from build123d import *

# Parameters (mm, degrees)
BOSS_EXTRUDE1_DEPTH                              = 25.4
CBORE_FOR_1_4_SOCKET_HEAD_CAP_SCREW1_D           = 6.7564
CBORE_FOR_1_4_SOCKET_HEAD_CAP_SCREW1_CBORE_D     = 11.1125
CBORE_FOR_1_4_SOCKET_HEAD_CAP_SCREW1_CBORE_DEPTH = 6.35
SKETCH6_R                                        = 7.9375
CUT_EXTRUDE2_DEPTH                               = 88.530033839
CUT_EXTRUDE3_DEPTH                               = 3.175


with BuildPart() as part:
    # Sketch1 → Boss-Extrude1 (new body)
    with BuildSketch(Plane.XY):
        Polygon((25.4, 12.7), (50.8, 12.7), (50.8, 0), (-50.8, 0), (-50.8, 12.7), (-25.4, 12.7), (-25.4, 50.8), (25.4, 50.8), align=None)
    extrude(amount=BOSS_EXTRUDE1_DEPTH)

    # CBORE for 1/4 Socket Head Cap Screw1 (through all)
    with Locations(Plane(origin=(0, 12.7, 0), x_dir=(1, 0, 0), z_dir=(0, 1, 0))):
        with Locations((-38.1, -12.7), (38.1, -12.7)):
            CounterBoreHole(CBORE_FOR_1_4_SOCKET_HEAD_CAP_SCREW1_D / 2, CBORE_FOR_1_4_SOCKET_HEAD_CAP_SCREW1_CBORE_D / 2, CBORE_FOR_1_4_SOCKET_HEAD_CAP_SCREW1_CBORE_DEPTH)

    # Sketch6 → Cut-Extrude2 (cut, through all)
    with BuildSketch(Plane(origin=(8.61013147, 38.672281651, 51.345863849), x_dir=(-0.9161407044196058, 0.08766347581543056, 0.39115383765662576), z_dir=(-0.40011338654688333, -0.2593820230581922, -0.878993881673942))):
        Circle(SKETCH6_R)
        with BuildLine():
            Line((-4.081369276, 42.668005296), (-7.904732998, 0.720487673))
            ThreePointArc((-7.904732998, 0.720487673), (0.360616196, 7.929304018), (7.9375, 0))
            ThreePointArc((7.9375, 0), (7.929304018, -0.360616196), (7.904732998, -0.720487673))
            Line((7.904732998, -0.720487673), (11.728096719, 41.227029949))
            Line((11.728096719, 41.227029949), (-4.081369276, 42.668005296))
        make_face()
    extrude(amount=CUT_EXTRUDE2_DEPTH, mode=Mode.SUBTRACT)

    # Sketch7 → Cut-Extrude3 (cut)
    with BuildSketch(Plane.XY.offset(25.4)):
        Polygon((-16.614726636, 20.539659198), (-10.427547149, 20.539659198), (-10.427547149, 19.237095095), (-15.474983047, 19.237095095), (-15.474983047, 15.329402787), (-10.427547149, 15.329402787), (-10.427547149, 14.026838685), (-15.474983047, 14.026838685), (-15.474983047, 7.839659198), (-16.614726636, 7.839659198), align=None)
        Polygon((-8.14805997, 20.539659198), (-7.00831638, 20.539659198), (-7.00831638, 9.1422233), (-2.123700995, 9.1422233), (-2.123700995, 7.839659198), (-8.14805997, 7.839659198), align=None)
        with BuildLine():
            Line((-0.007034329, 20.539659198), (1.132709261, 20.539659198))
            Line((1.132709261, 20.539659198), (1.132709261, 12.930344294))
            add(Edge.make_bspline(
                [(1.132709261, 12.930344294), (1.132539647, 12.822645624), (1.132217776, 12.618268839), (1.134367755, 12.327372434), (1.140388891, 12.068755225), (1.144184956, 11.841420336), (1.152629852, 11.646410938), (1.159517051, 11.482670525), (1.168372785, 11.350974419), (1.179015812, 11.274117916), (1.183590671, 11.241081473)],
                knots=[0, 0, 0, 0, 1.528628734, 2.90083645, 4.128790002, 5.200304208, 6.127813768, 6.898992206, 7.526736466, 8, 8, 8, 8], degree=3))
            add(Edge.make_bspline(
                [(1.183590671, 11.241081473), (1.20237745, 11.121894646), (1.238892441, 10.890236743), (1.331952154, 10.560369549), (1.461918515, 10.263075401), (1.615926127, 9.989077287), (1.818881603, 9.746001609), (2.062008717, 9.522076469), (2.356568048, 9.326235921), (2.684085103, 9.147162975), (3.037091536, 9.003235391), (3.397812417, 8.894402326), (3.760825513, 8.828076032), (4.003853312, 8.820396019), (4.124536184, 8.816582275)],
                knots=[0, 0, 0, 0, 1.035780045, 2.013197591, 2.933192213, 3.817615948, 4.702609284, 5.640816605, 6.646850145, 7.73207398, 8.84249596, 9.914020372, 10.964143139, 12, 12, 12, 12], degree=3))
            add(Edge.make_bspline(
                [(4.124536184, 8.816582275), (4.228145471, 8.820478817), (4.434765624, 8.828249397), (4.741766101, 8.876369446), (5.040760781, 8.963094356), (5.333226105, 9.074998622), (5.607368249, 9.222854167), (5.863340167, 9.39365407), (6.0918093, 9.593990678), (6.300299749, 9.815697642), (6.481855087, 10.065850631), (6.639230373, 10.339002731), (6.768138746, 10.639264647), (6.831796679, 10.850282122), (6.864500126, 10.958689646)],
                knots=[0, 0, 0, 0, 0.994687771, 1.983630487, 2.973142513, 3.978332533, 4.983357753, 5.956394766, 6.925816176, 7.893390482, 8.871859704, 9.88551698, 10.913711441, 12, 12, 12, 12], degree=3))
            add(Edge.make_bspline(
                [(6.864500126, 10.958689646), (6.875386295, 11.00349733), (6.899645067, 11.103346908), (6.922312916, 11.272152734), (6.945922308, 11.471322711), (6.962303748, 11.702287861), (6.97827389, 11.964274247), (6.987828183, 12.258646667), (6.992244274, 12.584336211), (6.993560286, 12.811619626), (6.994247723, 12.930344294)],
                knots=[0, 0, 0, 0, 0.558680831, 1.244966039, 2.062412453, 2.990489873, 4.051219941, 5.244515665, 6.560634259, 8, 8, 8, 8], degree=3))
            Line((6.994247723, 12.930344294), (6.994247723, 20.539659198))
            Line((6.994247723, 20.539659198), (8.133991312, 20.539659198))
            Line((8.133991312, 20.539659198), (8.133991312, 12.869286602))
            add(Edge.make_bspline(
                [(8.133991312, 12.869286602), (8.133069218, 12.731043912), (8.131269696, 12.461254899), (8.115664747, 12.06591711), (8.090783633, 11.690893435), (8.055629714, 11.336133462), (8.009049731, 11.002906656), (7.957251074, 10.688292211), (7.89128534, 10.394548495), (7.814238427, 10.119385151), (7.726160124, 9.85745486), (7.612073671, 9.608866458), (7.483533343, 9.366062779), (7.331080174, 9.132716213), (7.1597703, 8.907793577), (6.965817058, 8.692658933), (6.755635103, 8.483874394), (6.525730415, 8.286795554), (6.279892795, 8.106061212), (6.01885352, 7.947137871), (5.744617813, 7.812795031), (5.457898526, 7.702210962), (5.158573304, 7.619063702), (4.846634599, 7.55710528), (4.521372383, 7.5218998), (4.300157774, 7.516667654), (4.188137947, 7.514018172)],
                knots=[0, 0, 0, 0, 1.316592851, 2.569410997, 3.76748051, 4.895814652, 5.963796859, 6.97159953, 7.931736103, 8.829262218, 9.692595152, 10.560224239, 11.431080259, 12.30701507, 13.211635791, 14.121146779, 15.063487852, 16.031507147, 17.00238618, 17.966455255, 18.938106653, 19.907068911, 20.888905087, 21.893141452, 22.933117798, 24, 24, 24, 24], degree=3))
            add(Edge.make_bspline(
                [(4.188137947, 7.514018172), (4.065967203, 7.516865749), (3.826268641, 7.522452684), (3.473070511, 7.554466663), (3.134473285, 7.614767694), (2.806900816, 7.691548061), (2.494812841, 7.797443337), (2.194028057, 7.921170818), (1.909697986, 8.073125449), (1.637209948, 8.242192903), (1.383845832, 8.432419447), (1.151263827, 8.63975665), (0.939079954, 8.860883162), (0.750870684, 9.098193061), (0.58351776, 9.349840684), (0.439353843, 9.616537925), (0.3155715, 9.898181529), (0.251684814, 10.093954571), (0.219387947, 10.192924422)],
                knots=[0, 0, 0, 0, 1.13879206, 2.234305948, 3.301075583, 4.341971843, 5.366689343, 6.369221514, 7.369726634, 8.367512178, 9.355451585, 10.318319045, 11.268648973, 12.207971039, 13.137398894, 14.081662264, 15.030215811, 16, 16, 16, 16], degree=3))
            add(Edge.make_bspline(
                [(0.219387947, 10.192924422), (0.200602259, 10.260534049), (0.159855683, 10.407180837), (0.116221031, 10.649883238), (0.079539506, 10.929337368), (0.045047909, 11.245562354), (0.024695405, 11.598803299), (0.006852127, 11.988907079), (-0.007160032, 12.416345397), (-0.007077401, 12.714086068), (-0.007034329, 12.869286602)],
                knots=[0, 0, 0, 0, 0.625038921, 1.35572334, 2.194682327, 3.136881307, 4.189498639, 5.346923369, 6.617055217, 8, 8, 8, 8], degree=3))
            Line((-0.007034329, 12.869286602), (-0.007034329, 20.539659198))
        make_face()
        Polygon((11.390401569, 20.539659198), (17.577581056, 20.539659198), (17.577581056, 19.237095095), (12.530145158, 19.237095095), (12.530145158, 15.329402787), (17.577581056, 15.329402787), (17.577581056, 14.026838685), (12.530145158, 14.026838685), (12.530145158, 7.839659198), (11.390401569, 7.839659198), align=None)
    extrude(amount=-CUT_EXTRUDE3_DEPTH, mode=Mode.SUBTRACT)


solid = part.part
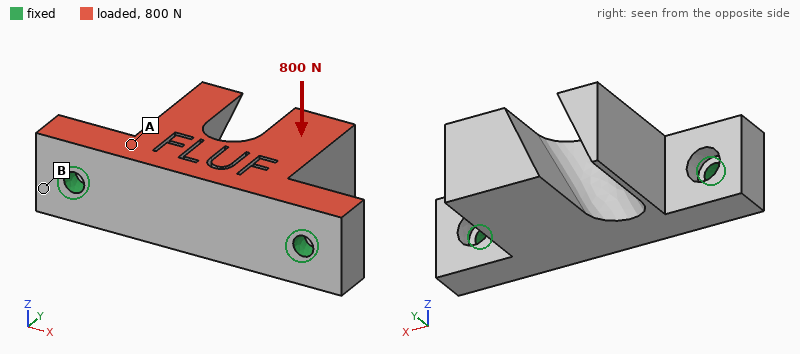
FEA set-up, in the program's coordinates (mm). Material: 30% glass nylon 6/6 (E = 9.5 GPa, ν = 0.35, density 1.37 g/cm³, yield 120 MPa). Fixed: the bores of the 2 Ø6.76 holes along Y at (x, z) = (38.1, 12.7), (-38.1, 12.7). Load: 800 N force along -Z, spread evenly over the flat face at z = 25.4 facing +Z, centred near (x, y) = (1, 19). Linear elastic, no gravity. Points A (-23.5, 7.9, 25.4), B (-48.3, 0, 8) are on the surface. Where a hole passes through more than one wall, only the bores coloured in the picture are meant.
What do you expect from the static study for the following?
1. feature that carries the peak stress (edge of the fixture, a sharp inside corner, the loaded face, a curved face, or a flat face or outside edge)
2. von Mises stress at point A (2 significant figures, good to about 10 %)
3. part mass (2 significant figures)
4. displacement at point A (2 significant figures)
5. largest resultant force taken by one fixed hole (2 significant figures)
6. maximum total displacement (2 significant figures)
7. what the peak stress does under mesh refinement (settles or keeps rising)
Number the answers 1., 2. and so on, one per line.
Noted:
1. edge of the fixture
2. 5.5 MPa
3. 91 g
4. 0.056 mm
5. 410 N
6. 0.23 mm
7. keeps rising
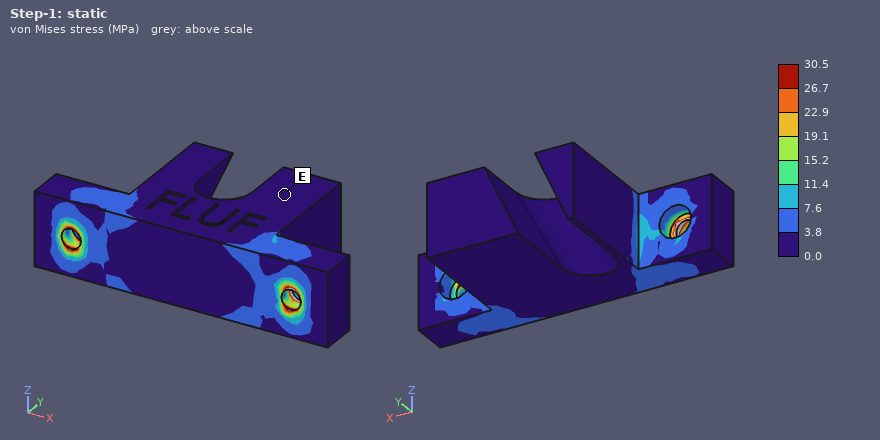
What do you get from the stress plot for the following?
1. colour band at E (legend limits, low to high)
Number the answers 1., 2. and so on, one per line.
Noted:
1. 0.0 to 3.8 MPa
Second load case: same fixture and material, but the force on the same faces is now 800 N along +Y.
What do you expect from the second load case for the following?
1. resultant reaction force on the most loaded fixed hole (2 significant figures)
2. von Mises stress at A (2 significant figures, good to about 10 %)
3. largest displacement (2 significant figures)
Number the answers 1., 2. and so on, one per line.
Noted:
1. 480 N
2. 3.6 MPa
3. 0.16 mm
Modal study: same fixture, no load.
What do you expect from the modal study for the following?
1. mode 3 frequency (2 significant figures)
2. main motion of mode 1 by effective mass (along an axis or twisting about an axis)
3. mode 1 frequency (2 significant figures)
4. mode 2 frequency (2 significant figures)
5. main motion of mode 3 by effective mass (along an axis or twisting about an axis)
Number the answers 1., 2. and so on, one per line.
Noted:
1. 3400 Hz
2. along Z
3. 1200 Hz
4. 3100 Hz
5. along Y
